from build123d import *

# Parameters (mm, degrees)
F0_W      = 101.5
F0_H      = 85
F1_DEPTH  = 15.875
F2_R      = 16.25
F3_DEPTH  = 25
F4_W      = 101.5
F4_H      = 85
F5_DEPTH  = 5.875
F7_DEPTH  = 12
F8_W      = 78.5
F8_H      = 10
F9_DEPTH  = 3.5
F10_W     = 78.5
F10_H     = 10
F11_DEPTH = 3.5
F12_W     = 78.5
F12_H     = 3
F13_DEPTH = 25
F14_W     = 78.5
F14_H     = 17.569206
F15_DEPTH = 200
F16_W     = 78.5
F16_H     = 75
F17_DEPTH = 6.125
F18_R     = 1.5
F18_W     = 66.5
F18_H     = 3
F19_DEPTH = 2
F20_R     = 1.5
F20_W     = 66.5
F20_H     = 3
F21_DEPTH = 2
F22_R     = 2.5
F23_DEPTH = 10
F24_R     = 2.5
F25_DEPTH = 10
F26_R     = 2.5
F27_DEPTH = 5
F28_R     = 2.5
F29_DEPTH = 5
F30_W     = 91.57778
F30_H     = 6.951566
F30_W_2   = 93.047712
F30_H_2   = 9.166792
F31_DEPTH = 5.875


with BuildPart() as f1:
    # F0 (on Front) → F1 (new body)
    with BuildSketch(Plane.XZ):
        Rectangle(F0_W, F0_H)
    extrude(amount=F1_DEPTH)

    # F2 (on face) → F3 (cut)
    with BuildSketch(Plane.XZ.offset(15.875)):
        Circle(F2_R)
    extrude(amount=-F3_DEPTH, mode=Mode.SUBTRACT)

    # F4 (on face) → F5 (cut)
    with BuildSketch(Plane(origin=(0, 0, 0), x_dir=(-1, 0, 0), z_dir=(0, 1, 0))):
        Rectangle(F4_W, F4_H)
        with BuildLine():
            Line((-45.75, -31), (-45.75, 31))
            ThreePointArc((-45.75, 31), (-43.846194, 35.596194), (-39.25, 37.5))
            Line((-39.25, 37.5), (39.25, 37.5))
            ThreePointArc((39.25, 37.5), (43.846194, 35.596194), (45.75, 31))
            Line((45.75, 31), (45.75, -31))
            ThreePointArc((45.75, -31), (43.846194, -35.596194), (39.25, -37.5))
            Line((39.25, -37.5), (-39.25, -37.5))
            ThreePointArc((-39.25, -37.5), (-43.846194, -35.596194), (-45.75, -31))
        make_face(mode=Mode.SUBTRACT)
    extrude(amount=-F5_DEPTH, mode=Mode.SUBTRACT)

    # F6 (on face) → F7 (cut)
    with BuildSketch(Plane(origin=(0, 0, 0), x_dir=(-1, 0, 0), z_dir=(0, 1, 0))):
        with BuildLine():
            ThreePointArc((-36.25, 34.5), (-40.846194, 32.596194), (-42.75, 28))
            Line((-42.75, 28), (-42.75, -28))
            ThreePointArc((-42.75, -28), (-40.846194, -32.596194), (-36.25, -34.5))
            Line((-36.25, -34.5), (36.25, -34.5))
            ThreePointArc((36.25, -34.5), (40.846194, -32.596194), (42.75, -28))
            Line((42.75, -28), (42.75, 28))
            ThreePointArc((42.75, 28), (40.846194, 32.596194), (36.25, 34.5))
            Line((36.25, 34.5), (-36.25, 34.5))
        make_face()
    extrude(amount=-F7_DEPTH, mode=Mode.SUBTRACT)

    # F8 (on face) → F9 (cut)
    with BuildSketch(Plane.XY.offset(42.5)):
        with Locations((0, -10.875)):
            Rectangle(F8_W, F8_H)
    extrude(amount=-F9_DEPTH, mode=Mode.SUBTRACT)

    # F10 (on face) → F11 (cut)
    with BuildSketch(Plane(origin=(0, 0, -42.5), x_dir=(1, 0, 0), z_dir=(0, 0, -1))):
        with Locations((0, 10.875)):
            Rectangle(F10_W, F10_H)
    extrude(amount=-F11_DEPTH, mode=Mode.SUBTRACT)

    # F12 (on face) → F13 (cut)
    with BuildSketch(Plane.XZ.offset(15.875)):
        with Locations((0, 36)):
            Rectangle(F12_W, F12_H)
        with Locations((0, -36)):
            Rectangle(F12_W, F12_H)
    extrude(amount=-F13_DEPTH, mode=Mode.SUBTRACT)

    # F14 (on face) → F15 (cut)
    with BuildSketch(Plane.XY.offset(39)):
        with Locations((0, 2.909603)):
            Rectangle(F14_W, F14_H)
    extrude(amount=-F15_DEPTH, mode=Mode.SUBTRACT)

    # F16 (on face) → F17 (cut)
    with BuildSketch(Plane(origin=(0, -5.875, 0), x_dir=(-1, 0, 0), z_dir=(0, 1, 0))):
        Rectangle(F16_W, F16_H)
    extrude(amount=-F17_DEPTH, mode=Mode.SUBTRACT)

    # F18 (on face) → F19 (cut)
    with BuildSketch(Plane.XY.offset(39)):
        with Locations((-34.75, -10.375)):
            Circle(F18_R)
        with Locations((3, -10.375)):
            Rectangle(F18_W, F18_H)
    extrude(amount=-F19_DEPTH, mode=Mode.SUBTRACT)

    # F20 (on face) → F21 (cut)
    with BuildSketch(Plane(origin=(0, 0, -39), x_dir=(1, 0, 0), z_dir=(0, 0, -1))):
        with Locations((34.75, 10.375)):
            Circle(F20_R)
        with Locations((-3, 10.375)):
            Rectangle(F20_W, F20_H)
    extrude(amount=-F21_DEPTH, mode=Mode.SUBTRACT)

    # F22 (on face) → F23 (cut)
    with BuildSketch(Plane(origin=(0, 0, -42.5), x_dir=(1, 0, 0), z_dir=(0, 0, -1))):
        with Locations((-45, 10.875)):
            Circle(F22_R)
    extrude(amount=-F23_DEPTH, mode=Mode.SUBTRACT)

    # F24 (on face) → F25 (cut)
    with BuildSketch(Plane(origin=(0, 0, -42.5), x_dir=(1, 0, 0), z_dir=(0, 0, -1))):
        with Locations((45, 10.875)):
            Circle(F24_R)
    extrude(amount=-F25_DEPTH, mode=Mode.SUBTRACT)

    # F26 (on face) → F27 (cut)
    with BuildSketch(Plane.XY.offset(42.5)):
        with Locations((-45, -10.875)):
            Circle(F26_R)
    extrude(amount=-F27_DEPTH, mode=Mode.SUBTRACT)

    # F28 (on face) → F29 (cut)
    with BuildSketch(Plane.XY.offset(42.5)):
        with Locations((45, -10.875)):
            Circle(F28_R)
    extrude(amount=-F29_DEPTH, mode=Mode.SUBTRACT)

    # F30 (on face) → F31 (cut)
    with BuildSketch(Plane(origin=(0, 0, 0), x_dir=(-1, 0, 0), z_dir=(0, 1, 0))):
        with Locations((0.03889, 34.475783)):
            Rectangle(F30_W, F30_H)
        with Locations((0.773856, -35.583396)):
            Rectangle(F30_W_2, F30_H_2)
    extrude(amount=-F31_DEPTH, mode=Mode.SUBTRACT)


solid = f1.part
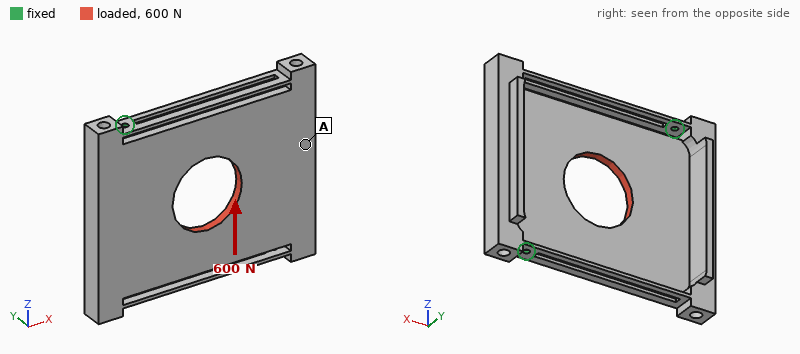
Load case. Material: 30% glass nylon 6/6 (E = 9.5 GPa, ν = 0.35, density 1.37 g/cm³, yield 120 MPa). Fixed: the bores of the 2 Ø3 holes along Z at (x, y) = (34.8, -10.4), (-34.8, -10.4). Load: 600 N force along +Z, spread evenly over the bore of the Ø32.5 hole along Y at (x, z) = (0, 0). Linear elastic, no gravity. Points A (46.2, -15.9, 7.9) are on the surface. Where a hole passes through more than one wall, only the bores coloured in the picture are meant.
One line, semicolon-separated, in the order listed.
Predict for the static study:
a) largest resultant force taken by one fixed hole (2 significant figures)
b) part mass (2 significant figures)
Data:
300 N; 52 g
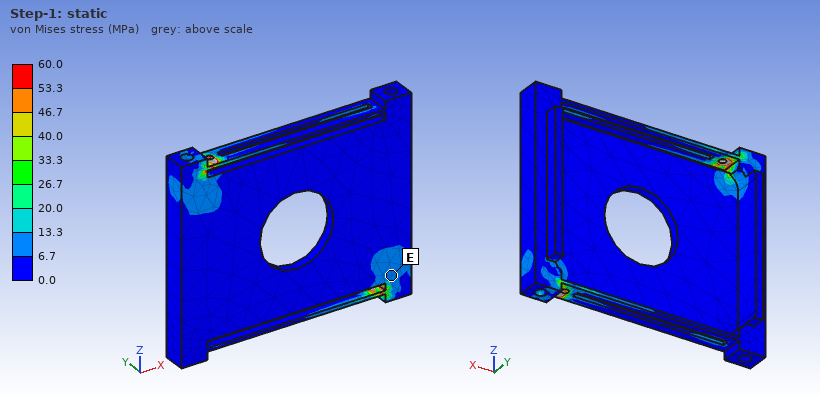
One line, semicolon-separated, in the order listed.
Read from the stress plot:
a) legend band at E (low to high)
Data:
6.7 to 13.3 MPa
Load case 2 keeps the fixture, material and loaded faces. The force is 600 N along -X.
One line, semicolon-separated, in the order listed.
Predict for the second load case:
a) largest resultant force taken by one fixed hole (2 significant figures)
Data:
300 N
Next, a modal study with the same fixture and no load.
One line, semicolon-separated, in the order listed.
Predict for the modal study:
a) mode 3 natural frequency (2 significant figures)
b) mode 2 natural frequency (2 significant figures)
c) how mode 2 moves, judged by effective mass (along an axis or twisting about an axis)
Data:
780 Hz; 310 Hz; along Y
